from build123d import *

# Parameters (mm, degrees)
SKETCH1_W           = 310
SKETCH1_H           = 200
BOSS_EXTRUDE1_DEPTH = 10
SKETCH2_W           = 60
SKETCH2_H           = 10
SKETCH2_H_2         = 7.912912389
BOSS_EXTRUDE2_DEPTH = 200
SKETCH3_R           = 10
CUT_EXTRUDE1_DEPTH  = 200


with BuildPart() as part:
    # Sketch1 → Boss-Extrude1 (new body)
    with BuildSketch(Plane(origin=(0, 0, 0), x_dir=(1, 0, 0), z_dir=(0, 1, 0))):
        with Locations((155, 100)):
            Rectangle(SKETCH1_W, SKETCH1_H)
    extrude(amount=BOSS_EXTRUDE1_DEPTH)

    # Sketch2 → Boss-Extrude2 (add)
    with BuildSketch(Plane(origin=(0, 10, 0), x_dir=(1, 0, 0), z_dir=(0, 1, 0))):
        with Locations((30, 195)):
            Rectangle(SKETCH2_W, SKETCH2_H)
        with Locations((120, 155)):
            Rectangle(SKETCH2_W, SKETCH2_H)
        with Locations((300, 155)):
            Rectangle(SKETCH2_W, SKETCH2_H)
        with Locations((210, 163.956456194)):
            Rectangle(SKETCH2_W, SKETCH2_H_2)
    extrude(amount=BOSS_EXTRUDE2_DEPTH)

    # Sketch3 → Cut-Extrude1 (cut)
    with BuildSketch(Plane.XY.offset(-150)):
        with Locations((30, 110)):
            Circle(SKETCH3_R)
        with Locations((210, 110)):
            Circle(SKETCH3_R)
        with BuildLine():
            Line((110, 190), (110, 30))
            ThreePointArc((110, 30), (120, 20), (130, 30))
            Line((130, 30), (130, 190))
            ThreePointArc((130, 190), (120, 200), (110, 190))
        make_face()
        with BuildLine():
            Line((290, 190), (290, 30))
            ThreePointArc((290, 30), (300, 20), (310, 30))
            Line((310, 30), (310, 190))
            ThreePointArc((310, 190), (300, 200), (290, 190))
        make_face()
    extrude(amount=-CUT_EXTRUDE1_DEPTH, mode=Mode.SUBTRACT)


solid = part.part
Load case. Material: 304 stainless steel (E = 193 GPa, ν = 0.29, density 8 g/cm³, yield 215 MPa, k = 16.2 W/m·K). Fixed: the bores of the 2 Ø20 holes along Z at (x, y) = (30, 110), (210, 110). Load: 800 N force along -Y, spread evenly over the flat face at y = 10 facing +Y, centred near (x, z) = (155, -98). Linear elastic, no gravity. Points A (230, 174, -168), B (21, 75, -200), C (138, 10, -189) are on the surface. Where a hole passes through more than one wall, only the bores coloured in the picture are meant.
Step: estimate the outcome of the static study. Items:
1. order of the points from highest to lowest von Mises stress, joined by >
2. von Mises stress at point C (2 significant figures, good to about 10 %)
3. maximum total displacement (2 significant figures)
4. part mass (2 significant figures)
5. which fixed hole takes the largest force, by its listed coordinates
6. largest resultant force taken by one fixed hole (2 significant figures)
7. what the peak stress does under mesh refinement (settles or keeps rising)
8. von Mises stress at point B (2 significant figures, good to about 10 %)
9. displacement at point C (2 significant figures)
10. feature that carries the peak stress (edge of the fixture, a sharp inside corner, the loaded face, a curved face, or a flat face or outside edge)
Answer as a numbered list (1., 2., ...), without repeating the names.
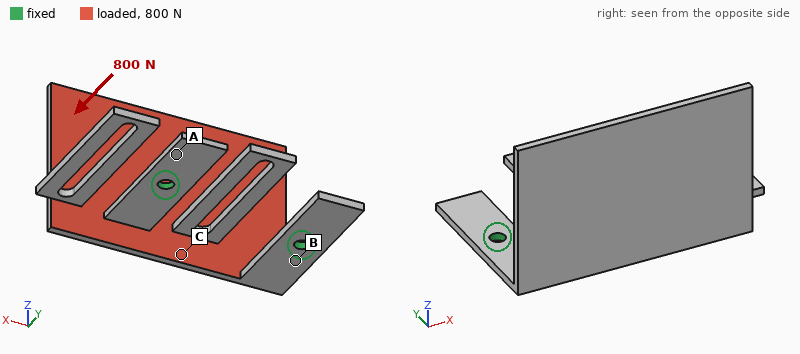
1. B > C > A
2. 9.1 MPa
3. 0.78 mm
4. 8.0 kg
5. (210, 110)
6. 920 N
7. keeps rising
8. 28 MPa
9. 0.17 mm
10. edge of the fixture
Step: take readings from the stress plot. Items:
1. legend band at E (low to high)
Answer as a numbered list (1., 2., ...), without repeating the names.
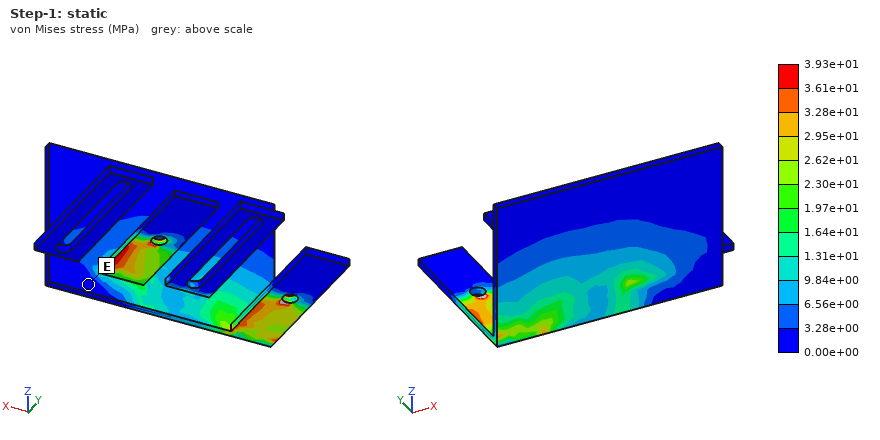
1. 0.00e+00 to 3.28e+00 MPa
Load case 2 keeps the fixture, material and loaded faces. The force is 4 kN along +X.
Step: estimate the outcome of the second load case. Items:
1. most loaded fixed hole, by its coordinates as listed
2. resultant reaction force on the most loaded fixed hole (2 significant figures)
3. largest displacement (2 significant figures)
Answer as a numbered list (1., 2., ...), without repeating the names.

1. (210, 110)
2. 3.9 kN
3. 0.88 mm
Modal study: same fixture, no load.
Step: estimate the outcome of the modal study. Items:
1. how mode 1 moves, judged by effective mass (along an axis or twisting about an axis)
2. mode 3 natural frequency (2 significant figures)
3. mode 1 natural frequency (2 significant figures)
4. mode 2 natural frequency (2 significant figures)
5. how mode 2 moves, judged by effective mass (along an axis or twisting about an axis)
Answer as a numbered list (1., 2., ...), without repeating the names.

1. along Y
2. 170 Hz
3. 76 Hz
4. 140 Hz
5. along Z
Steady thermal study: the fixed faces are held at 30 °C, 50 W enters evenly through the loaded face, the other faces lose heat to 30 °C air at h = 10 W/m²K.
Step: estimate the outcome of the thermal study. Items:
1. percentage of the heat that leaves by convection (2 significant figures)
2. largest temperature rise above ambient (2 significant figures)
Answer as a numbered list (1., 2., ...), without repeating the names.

1. 91 %
2. 56 K
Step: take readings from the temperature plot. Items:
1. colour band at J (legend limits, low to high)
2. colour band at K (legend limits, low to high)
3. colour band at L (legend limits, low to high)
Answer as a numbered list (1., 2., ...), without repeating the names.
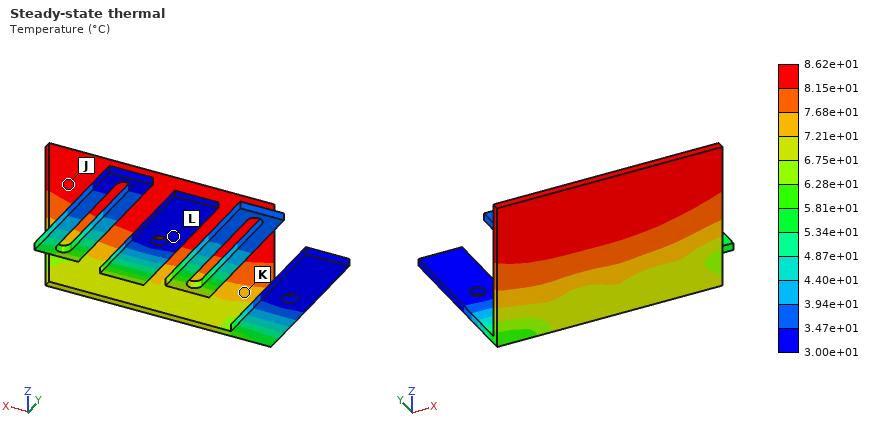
1. 8.15e+01 to 8.62e+01 °C
2. 7.21e+01 to 7.68e+01 °C
3. 3.00e+01 to 3.47e+01 °C
